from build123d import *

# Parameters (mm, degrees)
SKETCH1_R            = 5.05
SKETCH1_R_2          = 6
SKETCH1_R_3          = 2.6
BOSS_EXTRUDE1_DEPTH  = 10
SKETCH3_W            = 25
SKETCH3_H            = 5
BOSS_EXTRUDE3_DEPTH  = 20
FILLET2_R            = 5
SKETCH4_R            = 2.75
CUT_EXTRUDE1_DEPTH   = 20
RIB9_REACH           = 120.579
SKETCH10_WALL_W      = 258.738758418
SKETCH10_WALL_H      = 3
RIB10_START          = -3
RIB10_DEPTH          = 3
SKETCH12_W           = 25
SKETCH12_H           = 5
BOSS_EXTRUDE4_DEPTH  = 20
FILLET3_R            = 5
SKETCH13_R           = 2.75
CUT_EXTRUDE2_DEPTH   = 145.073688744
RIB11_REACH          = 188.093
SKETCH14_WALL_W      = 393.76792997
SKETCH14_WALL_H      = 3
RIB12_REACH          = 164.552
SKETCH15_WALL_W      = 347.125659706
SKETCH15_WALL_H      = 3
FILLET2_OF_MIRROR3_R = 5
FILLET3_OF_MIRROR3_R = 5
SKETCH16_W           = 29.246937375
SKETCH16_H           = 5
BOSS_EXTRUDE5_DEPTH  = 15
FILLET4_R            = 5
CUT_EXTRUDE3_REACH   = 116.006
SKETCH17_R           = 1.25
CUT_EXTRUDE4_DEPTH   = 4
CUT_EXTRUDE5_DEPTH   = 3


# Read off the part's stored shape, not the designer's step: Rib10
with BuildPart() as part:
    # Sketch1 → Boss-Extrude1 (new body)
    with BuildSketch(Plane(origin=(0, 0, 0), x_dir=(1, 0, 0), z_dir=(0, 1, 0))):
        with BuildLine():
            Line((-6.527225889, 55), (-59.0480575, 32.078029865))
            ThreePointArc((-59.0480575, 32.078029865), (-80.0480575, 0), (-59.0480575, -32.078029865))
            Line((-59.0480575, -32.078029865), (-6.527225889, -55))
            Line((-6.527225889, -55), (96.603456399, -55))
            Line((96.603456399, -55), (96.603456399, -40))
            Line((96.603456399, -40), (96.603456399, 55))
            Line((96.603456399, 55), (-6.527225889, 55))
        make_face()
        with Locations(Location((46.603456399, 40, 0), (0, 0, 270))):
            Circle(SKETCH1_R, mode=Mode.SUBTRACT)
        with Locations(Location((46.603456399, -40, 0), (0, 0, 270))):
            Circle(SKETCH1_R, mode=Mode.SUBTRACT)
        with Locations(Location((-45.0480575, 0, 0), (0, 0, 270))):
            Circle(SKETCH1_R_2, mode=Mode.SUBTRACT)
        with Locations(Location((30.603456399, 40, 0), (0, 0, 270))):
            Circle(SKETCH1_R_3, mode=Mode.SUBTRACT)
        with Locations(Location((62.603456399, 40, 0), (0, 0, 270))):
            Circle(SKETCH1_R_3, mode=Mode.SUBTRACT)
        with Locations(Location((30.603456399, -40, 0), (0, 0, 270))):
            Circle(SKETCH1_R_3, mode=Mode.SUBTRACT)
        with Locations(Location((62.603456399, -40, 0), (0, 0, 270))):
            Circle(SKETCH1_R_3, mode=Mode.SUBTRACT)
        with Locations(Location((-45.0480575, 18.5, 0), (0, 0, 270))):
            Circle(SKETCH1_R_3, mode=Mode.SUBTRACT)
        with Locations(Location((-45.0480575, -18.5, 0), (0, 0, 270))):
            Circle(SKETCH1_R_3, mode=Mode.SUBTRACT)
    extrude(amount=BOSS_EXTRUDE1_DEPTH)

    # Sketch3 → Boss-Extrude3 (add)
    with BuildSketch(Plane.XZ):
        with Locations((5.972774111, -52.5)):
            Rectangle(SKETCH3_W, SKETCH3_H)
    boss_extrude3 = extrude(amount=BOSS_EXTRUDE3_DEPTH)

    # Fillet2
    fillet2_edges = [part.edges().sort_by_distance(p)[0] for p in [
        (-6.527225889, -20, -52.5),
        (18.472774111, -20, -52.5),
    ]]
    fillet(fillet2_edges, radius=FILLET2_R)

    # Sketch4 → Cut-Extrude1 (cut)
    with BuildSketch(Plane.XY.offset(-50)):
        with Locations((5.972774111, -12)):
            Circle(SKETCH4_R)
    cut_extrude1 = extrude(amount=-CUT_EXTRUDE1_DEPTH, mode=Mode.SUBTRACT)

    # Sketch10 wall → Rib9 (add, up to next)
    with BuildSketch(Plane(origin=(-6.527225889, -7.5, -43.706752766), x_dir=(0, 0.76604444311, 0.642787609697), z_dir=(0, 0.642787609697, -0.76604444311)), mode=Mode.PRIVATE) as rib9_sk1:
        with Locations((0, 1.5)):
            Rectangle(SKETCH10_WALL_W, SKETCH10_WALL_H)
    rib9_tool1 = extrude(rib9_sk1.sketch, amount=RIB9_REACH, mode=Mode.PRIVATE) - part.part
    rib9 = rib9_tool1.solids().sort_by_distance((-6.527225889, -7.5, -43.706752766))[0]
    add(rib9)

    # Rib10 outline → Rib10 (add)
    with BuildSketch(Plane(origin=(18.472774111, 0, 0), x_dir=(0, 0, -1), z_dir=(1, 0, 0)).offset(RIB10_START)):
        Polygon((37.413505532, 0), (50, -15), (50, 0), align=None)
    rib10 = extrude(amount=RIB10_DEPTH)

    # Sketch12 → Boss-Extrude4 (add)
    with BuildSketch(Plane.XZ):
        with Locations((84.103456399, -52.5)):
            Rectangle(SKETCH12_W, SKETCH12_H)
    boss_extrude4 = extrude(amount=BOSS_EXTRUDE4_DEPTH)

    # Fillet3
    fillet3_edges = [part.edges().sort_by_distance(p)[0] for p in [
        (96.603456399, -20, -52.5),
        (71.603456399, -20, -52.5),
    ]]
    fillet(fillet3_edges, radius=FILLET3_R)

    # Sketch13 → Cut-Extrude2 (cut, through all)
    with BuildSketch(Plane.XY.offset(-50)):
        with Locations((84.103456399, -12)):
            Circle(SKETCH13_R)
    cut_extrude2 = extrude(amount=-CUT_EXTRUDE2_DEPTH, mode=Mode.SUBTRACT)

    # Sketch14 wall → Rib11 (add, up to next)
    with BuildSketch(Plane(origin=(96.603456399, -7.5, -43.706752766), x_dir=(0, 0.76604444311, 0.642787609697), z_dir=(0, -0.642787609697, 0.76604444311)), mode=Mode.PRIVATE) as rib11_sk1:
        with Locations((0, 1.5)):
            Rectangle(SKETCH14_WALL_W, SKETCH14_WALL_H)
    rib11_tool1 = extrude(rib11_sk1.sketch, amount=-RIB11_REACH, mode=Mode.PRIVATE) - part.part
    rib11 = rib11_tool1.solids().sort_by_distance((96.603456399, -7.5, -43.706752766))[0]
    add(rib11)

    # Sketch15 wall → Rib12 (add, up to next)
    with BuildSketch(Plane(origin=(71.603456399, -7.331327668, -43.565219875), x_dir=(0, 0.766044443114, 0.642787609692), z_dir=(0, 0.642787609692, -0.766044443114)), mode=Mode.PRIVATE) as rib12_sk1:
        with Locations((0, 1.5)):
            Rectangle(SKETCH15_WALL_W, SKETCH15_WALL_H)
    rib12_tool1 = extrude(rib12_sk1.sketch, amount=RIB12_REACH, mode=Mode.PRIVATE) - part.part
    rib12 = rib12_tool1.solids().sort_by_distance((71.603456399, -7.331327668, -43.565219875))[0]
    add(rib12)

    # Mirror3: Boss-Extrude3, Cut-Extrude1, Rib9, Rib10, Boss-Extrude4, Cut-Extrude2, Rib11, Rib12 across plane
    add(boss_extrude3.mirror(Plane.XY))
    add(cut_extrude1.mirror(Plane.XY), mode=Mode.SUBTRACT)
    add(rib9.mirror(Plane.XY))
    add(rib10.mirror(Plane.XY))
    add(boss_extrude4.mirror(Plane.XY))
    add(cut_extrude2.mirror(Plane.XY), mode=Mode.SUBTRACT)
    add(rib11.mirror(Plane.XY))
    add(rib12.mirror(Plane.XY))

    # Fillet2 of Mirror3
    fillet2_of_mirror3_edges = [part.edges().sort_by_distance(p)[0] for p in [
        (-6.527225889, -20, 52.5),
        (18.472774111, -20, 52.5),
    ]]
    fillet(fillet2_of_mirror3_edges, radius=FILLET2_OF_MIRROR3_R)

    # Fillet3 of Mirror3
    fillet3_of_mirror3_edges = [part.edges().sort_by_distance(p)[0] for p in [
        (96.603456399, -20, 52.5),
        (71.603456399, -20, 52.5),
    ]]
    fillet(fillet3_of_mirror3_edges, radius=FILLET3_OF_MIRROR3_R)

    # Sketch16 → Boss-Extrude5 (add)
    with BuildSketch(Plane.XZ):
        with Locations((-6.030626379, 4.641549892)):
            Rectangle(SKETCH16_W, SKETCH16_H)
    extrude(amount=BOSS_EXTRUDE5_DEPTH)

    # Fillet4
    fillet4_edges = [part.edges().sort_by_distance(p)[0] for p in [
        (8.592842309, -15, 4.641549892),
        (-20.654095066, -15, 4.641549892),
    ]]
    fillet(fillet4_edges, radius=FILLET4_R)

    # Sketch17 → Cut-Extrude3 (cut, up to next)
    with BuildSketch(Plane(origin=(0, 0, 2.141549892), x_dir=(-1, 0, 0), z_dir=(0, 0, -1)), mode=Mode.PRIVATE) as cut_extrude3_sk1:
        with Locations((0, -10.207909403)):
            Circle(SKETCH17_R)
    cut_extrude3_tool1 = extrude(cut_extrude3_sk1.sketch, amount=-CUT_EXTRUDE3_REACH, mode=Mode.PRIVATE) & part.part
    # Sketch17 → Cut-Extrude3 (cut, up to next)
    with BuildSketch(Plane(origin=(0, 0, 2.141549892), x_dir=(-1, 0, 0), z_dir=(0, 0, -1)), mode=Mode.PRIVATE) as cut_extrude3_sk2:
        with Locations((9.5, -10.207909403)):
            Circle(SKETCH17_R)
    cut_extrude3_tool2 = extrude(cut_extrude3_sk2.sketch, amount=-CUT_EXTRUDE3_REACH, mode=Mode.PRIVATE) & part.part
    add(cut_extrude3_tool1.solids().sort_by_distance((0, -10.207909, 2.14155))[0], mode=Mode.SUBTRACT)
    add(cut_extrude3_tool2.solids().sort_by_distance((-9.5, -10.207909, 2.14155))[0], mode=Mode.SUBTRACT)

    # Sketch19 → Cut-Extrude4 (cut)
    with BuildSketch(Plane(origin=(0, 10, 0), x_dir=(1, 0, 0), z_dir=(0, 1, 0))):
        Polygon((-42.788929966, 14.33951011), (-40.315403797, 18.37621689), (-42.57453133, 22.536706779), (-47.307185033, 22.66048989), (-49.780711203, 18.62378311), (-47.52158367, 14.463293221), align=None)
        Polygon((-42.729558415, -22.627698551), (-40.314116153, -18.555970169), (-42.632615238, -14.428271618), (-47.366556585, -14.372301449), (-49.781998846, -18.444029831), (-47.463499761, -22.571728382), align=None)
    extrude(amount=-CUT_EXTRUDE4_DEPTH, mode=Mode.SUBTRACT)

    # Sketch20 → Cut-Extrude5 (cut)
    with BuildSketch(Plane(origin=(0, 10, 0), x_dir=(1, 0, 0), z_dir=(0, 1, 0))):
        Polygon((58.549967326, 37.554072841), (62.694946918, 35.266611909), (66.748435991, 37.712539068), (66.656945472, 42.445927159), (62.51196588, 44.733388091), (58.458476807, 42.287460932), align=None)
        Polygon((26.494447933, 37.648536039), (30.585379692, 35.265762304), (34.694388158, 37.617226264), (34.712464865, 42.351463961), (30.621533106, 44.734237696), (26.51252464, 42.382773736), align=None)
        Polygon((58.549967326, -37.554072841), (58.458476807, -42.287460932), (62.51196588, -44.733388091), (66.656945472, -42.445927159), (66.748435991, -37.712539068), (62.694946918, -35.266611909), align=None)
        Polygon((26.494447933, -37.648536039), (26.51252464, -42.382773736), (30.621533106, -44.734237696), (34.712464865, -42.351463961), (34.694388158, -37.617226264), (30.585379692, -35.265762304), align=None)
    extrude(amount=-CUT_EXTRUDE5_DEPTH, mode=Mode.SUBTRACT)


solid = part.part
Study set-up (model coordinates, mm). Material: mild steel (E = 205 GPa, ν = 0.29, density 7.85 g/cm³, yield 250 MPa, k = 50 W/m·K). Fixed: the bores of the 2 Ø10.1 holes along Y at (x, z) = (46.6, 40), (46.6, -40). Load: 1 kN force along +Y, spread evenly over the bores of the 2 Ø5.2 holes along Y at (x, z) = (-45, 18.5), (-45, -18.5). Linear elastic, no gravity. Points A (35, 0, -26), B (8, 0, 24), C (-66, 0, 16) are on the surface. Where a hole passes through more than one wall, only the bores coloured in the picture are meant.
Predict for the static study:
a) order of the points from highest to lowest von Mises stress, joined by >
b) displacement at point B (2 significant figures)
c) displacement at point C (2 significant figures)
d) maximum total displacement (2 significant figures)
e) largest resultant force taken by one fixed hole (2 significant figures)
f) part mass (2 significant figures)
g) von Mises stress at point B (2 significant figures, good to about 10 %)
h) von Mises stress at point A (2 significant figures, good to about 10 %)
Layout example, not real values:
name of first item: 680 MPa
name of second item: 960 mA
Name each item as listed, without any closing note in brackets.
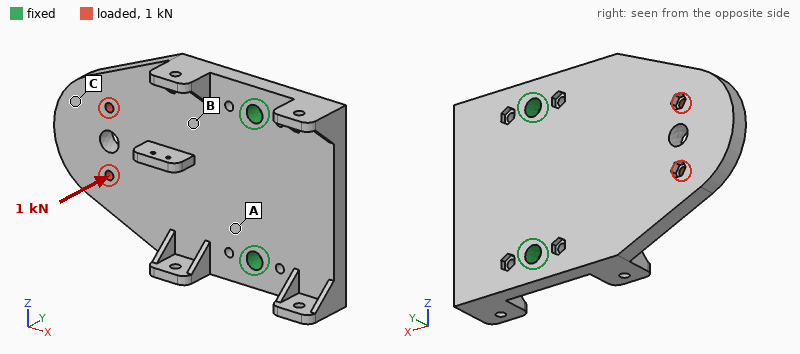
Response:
order of the points from highest to lowest von Mises stress, joined by >: A > B > C
displacement at point B: 0.042 mm
displacement at point C: 0.20 mm
maximum total displacement: 0.24 mm
largest resultant force taken by one fixed hole: 500 N
part mass: 1.4 kg
von Mises stress at point B: 24 MPa
von Mises stress at point A: 41 MPa
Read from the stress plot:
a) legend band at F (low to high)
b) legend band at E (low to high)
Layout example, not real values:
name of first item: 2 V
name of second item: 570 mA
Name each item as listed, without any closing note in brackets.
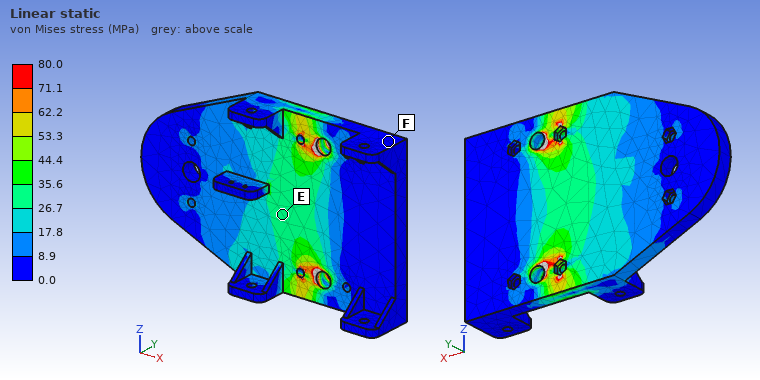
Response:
legend band at F: 0.0 to 8.9 MPa
legend band at E: 26.7 to 35.6 MPa
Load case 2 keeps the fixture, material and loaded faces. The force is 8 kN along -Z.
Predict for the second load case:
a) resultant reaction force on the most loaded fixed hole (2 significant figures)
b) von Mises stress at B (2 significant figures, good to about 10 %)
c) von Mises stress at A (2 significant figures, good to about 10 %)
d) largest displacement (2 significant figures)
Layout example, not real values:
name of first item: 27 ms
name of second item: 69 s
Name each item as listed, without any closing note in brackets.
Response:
resultant reaction force on the most loaded fixed hole: 9.6 kN
von Mises stress at B: 23 MPa
von Mises stress at A: 23 MPa
largest displacement: 31 µm
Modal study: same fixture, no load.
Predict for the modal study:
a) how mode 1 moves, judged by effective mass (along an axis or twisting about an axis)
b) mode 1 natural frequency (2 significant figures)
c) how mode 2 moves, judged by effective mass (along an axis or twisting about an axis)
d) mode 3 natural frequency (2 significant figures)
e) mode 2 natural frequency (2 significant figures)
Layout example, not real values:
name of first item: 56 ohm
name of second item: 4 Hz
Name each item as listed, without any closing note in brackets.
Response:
how mode 1 moves, judged by effective mass: along Y
mode 1 natural frequency: 650 Hz
how mode 2 moves, judged by effective mass: twisting about X
mode 3 natural frequency: 2600 Hz
mode 2 natural frequency: 2200 Hz
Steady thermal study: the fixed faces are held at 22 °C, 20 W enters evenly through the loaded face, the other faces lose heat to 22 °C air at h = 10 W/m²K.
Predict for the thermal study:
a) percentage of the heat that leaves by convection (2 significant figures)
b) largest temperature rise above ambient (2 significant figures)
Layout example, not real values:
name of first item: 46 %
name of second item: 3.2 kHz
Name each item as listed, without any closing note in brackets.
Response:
percentage of the heat that leaves by convection: 28 %
largest temperature rise above ambient: 39 K
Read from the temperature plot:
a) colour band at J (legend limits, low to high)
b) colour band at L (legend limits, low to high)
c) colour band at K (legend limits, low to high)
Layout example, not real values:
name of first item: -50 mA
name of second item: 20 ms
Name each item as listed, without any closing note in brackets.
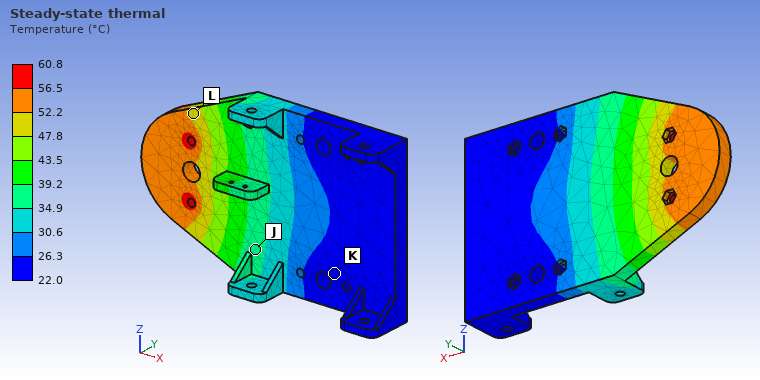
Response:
colour band at J: 34.9 to 39.2 °C
colour band at L: 47.8 to 52.2 °C
colour band at K: 22.0 to 26.3 °C
